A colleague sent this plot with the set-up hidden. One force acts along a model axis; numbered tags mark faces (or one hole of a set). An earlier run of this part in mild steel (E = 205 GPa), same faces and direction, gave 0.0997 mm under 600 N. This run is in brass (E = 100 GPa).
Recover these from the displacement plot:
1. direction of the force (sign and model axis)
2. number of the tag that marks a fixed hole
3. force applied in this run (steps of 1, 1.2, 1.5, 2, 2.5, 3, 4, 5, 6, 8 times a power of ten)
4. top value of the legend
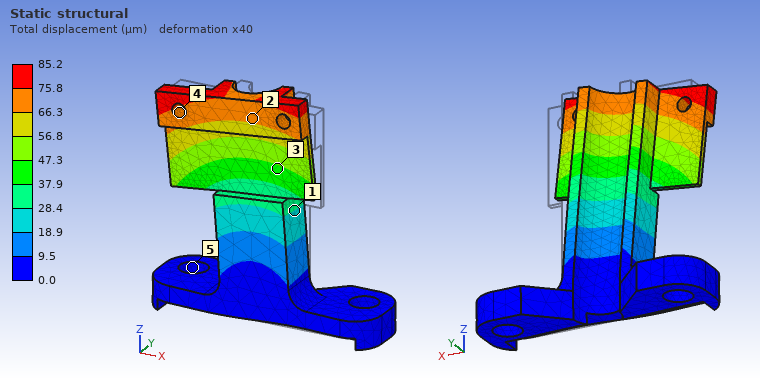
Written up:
-X
5
250 N
85.2 µm
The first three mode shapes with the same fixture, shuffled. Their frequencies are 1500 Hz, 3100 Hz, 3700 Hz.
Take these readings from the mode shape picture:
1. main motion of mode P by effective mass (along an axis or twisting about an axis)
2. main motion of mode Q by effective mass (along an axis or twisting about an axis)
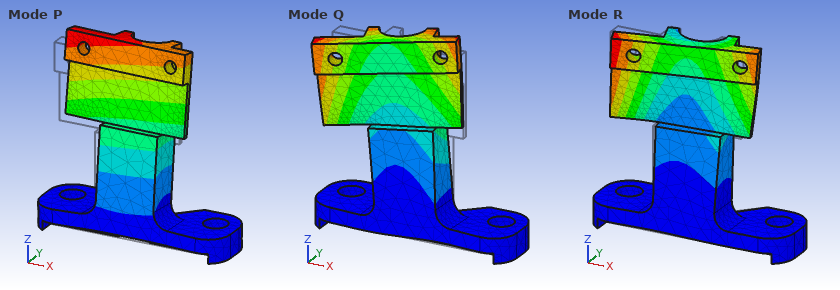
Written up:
along Y
along X
